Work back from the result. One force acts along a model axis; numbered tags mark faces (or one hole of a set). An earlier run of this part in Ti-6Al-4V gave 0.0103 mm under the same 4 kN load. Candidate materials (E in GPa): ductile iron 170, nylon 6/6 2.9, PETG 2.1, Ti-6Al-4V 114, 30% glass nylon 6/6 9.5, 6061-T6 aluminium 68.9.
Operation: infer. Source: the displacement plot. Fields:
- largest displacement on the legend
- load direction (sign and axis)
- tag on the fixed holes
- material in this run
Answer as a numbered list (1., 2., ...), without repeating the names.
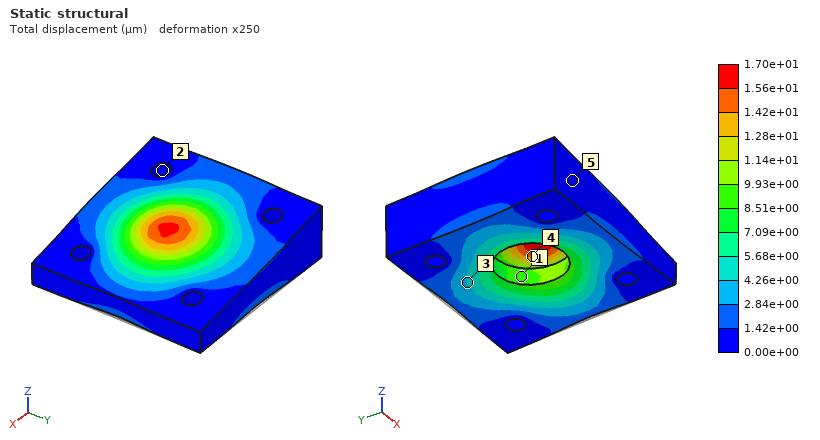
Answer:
1. 1.70e+01 µm
2. +Z
3. 2
4. 6061-T6 aluminium
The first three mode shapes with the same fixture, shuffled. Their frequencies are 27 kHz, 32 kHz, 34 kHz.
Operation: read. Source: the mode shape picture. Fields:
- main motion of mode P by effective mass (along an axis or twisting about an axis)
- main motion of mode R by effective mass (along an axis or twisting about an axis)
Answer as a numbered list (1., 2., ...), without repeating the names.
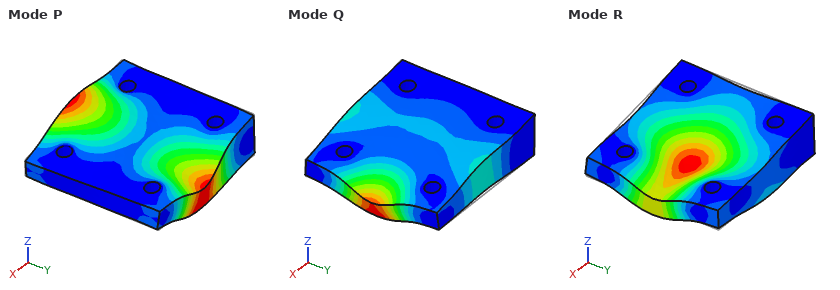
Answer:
1. twisting about X
2. along Z
